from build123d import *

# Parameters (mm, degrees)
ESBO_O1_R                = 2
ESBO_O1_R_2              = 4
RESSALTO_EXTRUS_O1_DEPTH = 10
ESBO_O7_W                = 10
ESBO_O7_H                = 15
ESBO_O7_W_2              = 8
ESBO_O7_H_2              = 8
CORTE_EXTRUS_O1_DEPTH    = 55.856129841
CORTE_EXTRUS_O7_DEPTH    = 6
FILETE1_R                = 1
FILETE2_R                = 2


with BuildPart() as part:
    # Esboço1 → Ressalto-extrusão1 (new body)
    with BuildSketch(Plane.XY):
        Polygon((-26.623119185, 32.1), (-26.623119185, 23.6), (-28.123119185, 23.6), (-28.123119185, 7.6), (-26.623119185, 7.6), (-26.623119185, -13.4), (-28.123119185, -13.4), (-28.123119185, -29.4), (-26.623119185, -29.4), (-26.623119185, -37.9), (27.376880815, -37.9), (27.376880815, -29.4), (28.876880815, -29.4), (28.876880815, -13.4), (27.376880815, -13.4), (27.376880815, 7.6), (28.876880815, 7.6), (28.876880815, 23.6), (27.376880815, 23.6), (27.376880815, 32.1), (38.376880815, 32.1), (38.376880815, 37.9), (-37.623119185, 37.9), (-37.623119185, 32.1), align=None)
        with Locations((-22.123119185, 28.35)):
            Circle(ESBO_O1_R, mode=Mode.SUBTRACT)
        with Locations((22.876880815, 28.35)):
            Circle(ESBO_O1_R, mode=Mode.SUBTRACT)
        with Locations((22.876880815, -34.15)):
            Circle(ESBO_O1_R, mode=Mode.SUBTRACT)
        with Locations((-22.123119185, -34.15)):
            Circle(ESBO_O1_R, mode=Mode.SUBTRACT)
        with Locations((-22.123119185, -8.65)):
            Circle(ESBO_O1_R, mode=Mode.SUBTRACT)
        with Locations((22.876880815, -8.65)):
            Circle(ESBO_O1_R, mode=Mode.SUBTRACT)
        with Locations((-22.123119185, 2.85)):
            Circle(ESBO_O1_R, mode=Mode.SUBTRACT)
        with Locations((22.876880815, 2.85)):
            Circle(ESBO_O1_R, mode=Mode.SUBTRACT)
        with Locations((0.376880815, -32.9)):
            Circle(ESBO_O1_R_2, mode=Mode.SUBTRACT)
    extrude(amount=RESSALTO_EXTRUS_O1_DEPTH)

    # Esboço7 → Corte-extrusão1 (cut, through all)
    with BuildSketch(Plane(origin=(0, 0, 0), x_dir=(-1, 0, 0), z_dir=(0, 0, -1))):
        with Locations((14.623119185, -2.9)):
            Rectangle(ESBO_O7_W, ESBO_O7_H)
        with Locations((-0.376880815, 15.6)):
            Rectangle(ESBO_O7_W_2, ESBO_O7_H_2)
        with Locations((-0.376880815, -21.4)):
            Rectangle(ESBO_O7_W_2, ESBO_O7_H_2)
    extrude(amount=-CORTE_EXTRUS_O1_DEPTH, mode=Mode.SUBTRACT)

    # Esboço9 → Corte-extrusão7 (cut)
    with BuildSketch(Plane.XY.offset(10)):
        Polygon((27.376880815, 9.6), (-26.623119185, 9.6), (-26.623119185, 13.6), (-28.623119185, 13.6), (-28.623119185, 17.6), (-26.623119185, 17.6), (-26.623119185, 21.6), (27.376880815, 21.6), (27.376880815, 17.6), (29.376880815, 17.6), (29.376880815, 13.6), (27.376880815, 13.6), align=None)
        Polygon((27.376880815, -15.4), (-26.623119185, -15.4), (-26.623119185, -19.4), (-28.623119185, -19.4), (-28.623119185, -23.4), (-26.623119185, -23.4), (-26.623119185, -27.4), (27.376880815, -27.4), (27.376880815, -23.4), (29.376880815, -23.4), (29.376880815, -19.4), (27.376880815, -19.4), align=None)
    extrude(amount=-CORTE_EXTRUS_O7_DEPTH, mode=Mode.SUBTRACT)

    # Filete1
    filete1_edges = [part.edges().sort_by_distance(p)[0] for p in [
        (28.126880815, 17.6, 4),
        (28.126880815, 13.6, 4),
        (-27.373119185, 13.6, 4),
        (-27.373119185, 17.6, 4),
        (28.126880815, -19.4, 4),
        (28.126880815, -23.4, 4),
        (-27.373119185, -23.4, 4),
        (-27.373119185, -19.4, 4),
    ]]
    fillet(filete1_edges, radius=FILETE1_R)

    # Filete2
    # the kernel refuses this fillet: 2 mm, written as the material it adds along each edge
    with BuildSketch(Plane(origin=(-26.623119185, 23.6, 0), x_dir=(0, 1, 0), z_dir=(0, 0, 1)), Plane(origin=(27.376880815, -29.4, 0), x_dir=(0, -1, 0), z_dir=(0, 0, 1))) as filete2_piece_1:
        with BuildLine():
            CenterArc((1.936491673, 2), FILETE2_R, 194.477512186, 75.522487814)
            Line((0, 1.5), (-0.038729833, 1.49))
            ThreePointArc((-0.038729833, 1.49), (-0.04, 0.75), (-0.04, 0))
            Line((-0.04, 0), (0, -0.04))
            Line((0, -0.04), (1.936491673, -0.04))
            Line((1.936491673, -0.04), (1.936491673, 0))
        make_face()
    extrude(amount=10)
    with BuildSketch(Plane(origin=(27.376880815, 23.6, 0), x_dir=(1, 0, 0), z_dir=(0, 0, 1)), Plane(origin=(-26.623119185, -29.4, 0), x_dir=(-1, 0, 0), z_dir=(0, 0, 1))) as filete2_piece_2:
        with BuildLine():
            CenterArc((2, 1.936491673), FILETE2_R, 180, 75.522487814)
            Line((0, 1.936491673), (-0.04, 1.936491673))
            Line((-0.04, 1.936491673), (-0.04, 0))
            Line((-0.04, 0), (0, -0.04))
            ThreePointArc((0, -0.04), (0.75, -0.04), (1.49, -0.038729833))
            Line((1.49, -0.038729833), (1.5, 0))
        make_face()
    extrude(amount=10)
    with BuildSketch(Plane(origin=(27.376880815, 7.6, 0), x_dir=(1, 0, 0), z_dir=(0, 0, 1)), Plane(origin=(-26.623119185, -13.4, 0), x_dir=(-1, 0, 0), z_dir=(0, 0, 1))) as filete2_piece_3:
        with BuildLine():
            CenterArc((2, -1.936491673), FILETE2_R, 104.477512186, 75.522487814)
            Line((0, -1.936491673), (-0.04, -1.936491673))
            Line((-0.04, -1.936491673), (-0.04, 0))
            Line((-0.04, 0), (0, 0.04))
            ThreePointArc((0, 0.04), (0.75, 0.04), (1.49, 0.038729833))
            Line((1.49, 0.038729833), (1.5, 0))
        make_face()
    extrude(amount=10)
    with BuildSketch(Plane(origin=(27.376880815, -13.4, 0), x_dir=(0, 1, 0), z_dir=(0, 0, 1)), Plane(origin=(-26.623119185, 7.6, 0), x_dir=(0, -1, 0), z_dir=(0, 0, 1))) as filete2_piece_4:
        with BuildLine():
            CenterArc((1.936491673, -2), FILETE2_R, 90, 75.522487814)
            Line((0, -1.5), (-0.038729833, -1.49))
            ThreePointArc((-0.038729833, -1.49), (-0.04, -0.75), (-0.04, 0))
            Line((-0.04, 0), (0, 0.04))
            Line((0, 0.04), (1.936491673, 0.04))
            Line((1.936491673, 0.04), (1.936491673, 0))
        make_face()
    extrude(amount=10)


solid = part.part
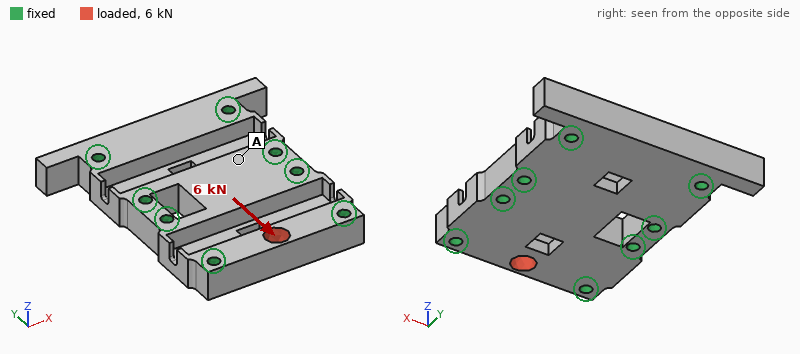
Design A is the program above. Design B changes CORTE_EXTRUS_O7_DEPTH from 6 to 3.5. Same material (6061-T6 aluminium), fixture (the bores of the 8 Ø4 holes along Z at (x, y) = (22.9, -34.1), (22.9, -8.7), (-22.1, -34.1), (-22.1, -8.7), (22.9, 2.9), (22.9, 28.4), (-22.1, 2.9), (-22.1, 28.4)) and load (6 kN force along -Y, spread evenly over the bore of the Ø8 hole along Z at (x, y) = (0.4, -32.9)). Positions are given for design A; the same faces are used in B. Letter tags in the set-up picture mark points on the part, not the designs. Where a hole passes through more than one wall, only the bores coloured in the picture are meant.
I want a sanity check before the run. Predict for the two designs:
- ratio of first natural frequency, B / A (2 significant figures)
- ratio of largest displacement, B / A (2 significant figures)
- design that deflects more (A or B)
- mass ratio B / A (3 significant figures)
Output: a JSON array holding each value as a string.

["0.99", "0.70", "A", "1.09"]
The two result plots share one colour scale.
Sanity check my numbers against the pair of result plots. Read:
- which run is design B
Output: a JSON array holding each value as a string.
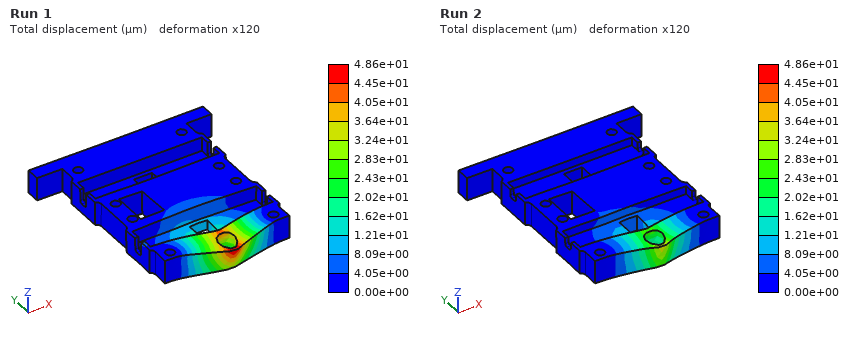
["Run 2"]
